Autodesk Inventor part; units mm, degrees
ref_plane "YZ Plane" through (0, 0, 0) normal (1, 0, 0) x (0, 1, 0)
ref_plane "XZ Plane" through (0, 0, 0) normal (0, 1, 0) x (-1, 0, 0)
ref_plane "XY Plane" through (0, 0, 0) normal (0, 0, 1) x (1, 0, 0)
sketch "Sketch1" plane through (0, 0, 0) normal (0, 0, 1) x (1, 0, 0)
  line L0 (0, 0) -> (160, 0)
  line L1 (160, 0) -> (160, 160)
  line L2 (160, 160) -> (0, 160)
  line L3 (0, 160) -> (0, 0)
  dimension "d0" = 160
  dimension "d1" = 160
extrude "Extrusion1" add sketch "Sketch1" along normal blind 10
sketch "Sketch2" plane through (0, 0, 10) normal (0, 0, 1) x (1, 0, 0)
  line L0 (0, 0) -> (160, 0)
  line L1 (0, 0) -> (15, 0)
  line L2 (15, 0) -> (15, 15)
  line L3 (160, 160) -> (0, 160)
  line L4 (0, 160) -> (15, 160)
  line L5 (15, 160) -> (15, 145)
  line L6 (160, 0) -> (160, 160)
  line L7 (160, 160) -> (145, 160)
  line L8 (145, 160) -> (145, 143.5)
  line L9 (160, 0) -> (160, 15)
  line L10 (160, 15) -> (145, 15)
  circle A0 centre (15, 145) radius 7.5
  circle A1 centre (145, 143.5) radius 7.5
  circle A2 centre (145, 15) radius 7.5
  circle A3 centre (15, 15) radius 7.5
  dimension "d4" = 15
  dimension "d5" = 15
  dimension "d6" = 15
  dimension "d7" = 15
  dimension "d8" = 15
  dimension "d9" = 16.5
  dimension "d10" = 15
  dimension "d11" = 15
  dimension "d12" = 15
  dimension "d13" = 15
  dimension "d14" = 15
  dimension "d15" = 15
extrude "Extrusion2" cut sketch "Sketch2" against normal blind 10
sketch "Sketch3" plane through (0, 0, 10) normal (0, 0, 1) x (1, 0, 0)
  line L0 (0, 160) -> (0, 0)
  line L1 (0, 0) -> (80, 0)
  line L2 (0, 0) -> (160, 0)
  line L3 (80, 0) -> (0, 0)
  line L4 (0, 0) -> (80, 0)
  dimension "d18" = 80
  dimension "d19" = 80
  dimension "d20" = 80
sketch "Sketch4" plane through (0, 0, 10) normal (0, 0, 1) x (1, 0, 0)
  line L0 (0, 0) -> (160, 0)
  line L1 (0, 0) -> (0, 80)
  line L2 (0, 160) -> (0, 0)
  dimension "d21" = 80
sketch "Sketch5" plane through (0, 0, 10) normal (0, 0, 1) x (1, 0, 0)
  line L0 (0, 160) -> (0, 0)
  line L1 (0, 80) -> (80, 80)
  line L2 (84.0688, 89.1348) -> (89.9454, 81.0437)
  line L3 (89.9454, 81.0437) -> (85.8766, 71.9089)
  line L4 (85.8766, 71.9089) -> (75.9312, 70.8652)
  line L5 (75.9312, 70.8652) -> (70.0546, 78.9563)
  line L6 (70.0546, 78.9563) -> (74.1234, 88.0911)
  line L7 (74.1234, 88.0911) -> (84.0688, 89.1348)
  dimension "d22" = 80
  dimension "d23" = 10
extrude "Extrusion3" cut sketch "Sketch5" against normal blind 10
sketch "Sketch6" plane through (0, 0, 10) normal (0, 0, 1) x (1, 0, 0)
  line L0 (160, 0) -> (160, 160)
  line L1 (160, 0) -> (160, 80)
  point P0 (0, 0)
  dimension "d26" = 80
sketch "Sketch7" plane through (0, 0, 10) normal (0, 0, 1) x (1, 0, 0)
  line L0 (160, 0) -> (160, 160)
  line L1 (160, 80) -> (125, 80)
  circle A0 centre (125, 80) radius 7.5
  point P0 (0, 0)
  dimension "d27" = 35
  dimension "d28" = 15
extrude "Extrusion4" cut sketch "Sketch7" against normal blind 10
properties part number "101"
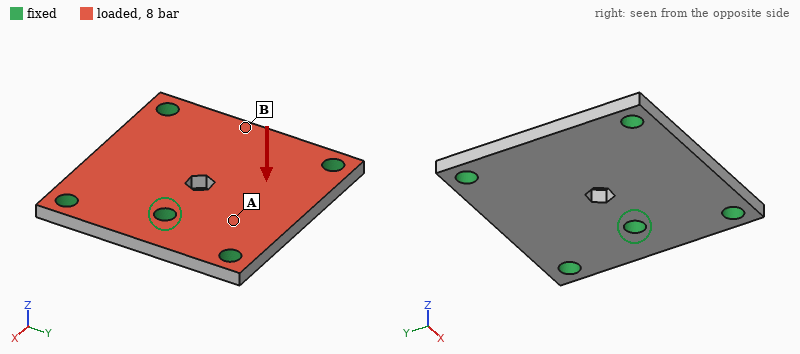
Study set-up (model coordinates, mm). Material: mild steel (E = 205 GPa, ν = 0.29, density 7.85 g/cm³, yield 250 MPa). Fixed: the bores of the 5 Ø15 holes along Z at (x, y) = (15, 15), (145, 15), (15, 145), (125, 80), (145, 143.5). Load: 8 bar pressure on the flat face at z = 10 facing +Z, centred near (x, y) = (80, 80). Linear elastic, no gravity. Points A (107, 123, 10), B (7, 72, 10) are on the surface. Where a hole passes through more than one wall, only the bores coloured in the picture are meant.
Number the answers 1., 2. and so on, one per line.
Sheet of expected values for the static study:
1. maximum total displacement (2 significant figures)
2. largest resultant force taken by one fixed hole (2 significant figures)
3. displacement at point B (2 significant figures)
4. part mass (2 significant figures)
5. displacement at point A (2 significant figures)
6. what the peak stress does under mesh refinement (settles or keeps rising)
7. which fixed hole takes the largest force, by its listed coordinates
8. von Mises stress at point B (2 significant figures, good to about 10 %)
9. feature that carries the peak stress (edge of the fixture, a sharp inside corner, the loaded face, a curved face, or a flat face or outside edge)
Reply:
1. 38 µm
2. 5.8 kN
3. 29 µm
4. 1.9 kg
5. 16 µm
6. keeps rising
7. (125, 80)
8. 30 MPa
9. edge of the fixture
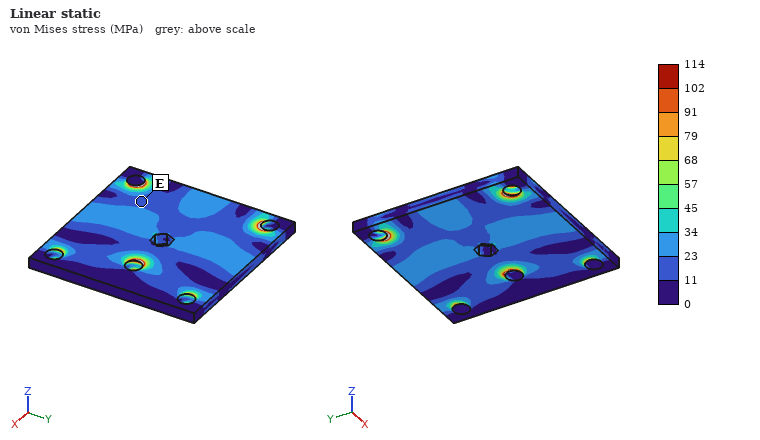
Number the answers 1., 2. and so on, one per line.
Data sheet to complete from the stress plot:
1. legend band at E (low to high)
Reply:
1. 11 to 23 MPa
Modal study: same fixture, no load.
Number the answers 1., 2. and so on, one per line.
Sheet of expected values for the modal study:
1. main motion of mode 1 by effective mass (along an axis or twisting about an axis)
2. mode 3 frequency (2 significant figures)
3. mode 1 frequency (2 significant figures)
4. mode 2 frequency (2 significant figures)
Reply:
1. along Z
2. 3900 Hz
3. 3100 Hz
4. 3800 Hz
